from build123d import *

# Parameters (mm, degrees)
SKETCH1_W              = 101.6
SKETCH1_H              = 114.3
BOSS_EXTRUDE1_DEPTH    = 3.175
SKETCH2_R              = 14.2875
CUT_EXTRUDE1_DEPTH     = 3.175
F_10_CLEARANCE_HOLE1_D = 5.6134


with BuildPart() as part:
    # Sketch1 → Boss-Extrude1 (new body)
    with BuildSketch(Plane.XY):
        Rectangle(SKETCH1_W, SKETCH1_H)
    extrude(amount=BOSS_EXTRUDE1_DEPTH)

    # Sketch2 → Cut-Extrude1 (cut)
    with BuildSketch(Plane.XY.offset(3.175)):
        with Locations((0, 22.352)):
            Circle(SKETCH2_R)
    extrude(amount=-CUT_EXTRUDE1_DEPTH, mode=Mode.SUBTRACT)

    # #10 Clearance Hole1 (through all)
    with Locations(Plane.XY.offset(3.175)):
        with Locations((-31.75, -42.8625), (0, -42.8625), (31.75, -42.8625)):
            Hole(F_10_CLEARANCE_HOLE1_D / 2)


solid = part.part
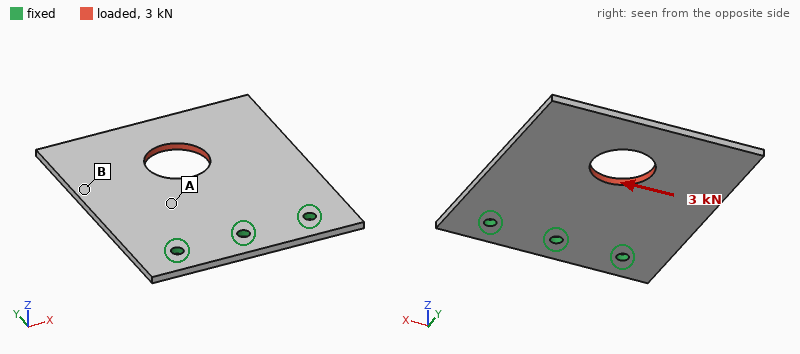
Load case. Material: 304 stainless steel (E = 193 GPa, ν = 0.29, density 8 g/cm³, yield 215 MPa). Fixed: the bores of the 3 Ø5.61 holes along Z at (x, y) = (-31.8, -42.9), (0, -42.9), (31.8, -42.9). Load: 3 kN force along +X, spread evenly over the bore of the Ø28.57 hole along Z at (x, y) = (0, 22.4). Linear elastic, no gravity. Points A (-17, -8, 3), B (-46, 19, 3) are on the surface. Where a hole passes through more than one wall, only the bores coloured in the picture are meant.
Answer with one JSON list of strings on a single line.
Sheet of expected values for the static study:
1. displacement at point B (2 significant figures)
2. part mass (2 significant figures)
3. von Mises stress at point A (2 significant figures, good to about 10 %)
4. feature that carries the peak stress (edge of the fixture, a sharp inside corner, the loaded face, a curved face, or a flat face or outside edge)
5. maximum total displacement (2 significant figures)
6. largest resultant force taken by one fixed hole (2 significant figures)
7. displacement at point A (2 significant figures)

["22 µm", "280 g", "21 MPa", "edge of the fixture", "33 µm", "3.1 kN", "10.0 µm"]
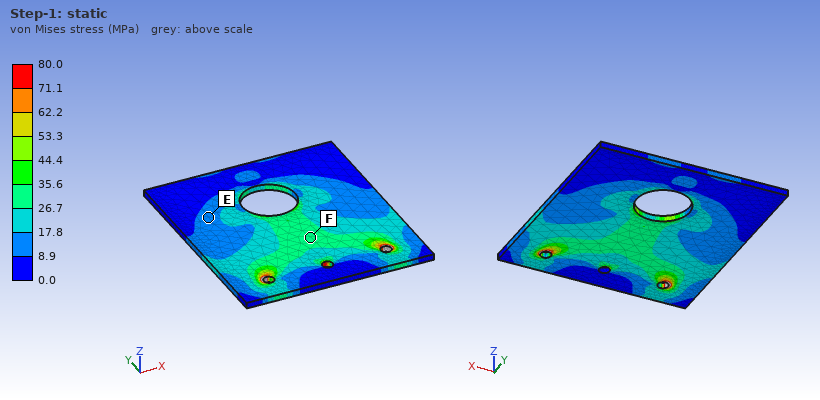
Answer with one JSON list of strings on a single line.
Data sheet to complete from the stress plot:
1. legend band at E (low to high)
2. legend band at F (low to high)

["8.9 to 17.8 MPa", "26.7 to 35.6 MPa"]
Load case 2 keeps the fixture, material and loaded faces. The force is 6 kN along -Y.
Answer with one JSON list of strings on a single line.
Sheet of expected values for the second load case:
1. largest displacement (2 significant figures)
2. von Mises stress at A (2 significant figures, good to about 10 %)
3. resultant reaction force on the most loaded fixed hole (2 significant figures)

["14 µm", "26 MPa", "2.1 kN"]
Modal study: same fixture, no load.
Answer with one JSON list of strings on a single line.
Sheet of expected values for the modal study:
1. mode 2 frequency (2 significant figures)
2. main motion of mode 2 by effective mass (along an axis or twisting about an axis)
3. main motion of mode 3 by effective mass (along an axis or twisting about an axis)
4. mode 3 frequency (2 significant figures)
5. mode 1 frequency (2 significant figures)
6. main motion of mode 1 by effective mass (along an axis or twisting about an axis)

["590 Hz", "twisting about Y", "along Z", "1500 Hz", "260 Hz", "along Z"]
